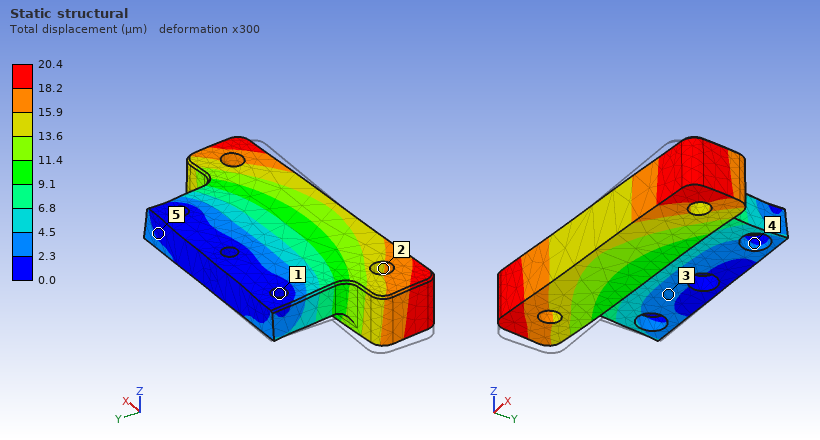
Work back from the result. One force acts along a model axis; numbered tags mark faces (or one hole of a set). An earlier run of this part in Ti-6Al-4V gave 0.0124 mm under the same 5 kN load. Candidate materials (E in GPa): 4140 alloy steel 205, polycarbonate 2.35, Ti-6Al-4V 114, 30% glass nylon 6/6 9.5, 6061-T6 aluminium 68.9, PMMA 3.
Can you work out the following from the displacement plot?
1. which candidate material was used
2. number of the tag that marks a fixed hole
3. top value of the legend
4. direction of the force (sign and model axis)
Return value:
6061-T6 aluminium
1
20.4 µm
+X
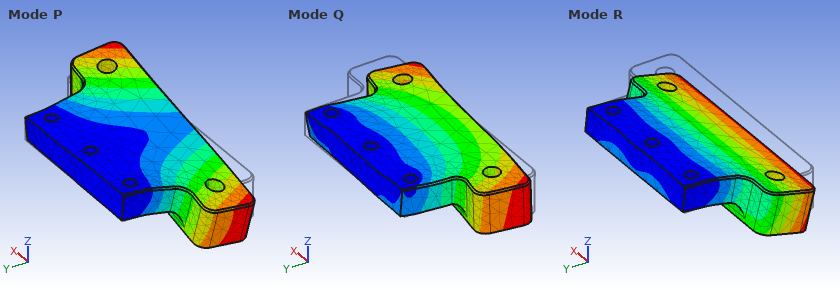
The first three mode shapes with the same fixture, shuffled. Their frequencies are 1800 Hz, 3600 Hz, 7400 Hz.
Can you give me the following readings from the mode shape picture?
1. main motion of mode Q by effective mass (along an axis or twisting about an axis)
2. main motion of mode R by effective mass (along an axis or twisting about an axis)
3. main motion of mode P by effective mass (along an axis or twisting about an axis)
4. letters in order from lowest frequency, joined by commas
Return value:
along X
along Z
twisting about Y
R, P, Q
